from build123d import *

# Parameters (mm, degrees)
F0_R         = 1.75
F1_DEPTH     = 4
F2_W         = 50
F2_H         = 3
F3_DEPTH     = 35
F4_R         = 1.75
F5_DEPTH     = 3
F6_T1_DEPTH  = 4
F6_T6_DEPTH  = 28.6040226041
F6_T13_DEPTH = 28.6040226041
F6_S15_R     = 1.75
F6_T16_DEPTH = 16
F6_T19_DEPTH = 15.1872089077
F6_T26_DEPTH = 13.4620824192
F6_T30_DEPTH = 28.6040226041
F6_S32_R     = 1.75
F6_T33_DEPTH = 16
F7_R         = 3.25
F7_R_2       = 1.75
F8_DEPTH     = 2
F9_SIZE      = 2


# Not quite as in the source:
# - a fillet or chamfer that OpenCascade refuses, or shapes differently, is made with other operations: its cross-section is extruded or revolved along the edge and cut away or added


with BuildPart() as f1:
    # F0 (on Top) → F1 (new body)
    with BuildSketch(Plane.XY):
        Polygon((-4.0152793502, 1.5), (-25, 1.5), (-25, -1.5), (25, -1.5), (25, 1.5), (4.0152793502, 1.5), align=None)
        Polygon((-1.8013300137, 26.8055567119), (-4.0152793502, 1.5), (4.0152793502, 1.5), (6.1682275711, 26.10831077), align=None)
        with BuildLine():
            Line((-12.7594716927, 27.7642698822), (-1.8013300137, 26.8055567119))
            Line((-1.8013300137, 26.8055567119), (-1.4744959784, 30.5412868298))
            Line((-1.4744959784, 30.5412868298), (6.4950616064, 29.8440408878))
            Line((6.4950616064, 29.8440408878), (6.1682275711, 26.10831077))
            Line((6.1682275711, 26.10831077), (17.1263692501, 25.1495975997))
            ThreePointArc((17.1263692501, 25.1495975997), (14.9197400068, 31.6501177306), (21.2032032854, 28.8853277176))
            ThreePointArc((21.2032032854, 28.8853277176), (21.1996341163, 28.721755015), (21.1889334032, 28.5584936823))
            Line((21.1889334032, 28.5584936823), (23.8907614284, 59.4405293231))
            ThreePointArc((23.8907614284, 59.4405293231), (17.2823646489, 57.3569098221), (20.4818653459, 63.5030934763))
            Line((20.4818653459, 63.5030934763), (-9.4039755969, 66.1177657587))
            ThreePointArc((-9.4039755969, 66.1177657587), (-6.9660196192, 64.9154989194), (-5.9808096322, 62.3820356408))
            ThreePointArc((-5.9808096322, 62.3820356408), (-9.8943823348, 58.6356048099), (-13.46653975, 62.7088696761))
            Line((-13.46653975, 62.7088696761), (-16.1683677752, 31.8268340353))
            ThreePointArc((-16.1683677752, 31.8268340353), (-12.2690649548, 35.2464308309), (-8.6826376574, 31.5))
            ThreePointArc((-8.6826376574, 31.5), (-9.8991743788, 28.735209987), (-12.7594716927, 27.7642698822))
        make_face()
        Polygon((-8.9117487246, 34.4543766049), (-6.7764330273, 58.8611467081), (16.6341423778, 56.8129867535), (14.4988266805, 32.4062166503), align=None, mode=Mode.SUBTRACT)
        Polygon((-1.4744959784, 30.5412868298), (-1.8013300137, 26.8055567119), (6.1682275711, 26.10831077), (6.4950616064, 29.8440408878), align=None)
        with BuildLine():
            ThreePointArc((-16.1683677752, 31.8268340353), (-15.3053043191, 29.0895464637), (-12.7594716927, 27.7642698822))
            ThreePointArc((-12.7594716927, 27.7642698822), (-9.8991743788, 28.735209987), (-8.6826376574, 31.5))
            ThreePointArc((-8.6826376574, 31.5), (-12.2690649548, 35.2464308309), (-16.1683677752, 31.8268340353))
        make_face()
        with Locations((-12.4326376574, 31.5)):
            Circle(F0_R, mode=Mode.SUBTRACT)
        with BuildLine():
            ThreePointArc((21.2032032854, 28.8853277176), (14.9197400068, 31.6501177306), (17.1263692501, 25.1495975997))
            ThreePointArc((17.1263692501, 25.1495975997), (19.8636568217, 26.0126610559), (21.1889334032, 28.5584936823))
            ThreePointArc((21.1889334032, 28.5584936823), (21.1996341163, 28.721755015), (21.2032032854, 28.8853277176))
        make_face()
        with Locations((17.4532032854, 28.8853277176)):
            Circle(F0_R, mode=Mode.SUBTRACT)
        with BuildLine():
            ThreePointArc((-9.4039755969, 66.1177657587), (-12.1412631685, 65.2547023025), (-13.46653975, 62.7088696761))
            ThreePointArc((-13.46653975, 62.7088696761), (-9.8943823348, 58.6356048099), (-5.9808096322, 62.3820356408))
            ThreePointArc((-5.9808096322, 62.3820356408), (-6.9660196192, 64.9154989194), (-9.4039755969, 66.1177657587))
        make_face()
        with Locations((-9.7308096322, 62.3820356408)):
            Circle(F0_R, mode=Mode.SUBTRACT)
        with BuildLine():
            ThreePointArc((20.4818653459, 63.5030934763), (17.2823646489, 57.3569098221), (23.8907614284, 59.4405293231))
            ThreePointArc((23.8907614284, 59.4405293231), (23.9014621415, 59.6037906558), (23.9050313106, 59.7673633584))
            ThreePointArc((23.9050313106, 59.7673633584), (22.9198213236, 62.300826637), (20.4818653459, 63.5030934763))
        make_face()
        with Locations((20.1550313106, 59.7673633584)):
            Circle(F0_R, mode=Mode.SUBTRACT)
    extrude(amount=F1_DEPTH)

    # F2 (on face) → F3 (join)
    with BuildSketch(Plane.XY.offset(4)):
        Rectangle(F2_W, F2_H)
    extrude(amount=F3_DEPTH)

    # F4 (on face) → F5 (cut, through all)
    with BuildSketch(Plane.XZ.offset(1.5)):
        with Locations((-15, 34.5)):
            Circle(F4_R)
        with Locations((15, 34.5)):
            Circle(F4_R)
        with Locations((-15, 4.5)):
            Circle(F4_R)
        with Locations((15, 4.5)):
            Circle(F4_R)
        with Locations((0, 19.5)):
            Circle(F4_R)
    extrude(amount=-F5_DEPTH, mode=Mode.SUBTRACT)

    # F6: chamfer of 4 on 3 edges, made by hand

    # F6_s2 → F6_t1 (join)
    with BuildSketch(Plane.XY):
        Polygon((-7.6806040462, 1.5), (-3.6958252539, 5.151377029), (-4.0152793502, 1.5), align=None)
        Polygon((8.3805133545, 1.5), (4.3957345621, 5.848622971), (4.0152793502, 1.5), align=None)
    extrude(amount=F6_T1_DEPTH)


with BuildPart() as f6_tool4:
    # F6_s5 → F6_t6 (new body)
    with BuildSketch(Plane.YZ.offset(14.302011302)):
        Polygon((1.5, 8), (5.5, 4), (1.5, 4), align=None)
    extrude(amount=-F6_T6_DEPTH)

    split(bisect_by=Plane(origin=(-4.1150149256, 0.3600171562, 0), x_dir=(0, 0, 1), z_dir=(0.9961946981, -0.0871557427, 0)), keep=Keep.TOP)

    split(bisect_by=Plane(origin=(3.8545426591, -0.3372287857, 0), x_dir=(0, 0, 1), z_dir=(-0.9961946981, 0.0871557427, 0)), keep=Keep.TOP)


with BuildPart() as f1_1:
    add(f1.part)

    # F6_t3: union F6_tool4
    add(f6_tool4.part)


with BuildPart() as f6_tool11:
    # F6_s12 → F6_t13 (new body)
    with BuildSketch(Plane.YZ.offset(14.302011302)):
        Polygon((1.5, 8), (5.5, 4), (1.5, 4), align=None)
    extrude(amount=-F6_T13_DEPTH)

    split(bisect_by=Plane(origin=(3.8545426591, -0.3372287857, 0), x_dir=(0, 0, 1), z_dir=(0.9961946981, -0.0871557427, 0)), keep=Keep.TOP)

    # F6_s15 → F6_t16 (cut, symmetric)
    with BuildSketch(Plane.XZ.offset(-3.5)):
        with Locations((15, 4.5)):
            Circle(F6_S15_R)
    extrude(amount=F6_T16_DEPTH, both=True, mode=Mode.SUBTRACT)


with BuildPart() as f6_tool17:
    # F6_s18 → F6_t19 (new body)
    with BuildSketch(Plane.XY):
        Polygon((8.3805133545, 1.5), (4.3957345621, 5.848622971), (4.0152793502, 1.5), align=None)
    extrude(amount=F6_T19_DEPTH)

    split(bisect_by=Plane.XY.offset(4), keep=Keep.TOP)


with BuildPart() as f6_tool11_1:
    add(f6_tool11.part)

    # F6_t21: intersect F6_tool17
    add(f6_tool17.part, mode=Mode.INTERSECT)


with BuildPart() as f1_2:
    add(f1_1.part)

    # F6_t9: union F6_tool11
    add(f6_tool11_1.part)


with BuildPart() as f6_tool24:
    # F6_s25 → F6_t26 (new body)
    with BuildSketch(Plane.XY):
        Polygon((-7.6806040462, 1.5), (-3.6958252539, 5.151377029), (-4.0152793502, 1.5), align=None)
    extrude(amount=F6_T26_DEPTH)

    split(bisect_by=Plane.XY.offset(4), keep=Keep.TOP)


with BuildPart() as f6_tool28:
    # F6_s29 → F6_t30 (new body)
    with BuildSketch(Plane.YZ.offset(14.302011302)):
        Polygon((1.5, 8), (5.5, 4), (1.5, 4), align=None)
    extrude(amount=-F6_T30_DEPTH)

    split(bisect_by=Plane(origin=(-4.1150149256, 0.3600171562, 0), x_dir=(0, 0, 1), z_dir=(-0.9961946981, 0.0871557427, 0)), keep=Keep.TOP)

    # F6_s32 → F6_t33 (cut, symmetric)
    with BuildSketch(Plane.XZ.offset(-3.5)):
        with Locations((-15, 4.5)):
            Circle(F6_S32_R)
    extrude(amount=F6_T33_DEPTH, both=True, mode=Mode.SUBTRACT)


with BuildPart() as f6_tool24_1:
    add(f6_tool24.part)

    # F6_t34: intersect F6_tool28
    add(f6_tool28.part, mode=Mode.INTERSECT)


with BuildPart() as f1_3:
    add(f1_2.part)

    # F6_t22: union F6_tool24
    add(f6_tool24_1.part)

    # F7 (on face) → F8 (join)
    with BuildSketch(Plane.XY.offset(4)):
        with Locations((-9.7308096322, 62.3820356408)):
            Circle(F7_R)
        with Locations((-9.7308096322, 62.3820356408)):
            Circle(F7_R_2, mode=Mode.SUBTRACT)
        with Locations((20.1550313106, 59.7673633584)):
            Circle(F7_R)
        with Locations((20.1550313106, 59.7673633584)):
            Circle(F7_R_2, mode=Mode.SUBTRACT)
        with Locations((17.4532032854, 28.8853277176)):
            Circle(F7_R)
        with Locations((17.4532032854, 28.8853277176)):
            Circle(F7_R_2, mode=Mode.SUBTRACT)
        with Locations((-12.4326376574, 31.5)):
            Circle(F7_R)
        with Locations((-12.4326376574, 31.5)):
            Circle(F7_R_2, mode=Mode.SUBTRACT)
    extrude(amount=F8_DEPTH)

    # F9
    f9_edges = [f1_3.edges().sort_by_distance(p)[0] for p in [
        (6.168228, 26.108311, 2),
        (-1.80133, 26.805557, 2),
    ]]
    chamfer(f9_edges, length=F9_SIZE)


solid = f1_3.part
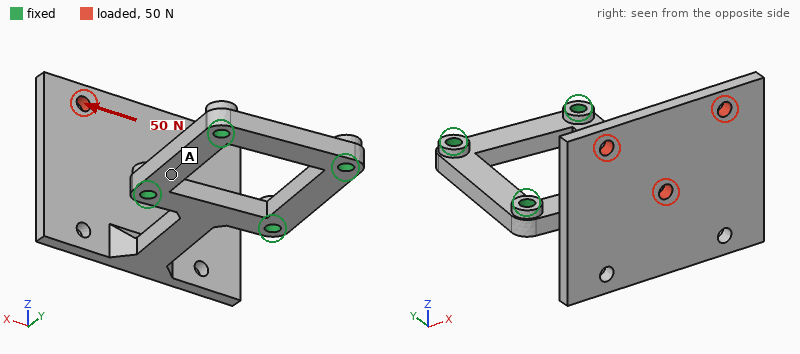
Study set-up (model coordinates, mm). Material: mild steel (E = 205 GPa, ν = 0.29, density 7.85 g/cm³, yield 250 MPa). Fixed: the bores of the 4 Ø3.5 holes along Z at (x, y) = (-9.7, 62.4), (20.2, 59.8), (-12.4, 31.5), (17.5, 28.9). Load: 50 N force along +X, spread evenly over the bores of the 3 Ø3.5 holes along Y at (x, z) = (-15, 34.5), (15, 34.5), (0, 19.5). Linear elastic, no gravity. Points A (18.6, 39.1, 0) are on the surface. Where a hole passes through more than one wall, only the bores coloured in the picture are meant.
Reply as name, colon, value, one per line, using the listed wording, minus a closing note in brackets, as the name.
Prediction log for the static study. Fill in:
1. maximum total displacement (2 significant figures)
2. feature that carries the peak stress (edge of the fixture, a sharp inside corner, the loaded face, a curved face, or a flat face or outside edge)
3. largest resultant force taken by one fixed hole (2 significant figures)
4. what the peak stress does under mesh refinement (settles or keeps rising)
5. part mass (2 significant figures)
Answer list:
maximum total displacement: 0.17 mm
feature that carries the peak stress: a sharp inside corner
largest resultant force taken by one fixed hole: 100 N
what the peak stress does under mesh refinement: keeps rising
part mass: 80 g
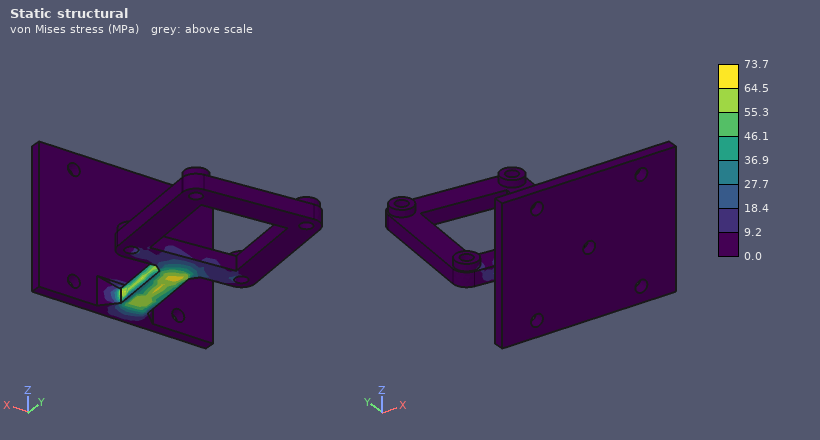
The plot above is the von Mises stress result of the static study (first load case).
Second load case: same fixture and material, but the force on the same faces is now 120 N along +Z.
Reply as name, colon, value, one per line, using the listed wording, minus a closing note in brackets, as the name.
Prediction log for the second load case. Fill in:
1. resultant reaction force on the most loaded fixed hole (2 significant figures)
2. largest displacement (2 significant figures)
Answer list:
resultant reaction force on the most loaded fixed hole: 66 N
largest displacement: 0.34 mm
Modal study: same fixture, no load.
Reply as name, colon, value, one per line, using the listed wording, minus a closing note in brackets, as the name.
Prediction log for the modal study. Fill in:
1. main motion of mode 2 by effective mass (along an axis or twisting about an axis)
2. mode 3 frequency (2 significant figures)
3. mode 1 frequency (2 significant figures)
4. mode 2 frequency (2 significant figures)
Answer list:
main motion of mode 2 by effective mass: along X
mode 3 frequency: 1300 Hz
mode 1 frequency: 440 Hz
mode 2 frequency: 570 Hz
